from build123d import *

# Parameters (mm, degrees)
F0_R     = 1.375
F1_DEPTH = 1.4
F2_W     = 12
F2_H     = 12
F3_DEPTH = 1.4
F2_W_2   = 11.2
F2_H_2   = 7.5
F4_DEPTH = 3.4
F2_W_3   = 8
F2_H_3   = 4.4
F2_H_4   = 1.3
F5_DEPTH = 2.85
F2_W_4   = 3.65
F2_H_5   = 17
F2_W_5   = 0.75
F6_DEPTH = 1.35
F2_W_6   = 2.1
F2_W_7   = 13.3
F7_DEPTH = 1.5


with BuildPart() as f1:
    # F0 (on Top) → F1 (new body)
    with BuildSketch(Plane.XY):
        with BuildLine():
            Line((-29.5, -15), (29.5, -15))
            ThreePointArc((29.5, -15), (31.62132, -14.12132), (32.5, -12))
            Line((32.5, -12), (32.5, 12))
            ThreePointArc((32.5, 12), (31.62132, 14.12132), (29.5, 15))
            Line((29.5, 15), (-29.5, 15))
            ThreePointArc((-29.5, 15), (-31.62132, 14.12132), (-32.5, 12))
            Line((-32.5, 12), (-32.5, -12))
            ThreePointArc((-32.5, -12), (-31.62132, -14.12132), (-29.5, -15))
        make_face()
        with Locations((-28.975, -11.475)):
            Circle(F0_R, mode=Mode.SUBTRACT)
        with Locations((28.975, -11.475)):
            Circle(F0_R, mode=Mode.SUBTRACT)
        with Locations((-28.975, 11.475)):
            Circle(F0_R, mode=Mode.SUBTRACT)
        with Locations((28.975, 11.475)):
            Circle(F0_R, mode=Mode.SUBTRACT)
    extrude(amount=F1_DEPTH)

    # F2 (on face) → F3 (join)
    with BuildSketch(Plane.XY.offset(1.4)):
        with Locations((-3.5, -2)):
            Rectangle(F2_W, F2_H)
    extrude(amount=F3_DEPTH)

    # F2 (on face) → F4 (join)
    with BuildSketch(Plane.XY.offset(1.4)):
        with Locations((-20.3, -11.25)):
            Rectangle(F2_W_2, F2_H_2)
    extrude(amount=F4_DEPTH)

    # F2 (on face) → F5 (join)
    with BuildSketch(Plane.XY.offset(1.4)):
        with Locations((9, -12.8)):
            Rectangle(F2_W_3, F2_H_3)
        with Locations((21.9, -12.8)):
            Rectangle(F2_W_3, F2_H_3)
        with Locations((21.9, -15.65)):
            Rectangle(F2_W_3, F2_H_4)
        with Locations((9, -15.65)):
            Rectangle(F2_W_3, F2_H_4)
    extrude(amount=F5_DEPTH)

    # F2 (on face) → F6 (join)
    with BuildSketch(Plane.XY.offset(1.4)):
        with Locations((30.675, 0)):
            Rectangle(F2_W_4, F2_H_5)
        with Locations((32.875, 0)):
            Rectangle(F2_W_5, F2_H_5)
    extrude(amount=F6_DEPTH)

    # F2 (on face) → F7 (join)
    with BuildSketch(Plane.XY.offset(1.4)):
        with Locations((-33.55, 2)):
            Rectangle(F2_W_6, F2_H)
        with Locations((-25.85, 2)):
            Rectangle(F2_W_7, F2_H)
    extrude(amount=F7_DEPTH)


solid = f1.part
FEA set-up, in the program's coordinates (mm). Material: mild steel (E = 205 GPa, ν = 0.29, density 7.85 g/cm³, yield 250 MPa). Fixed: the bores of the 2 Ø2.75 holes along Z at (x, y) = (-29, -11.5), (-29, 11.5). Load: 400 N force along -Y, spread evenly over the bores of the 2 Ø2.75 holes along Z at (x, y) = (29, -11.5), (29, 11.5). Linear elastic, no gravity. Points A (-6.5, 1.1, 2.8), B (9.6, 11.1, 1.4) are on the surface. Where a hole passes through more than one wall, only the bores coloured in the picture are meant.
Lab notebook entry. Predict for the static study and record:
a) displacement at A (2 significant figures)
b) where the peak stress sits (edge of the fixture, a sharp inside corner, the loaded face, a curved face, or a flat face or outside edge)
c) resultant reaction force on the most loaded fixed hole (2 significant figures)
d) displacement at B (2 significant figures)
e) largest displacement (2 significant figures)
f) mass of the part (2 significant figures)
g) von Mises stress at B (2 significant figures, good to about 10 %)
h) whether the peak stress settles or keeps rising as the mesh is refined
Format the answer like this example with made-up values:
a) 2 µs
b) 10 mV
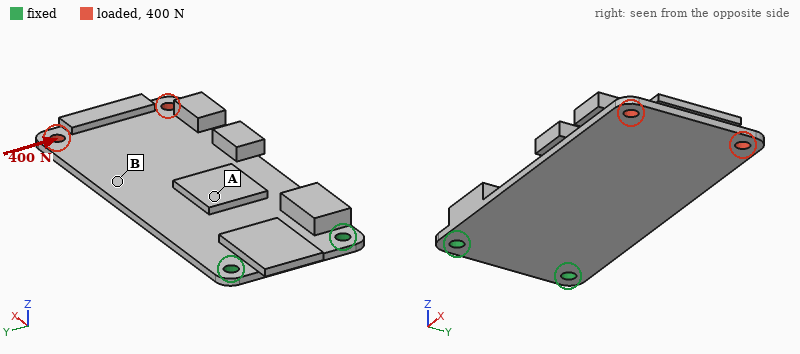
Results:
a) 12 µm
b) edge of the fixture
c) 1.0 kN
d) 34 µm
e) 66 µm
f) 30 g
g) 29 MPa
h) keeps rising
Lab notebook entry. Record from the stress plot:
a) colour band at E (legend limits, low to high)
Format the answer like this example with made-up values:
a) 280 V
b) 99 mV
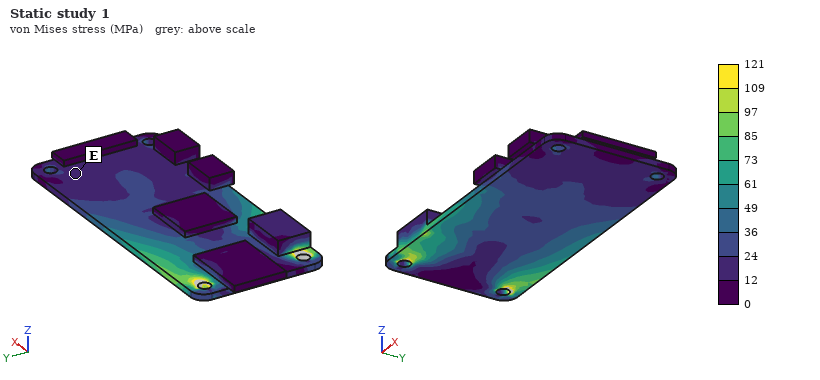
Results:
a) 12 to 24 MPa
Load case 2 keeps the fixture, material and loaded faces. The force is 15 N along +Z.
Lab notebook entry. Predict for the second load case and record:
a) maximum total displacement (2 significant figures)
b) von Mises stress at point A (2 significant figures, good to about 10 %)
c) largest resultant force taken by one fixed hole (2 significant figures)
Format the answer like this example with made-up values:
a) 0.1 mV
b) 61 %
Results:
a) 0.44 mm
b) 25 MPa
c) 13 N
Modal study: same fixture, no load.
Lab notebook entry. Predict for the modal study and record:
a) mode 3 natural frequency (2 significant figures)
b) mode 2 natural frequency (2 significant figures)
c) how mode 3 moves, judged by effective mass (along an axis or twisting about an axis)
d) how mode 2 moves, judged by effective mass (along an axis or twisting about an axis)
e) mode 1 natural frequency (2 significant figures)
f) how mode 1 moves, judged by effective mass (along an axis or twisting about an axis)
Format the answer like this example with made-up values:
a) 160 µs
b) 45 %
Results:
a) 2000 Hz
b) 1600 Hz
c) along Z
d) twisting about X
e) 360 Hz
f) along Z
